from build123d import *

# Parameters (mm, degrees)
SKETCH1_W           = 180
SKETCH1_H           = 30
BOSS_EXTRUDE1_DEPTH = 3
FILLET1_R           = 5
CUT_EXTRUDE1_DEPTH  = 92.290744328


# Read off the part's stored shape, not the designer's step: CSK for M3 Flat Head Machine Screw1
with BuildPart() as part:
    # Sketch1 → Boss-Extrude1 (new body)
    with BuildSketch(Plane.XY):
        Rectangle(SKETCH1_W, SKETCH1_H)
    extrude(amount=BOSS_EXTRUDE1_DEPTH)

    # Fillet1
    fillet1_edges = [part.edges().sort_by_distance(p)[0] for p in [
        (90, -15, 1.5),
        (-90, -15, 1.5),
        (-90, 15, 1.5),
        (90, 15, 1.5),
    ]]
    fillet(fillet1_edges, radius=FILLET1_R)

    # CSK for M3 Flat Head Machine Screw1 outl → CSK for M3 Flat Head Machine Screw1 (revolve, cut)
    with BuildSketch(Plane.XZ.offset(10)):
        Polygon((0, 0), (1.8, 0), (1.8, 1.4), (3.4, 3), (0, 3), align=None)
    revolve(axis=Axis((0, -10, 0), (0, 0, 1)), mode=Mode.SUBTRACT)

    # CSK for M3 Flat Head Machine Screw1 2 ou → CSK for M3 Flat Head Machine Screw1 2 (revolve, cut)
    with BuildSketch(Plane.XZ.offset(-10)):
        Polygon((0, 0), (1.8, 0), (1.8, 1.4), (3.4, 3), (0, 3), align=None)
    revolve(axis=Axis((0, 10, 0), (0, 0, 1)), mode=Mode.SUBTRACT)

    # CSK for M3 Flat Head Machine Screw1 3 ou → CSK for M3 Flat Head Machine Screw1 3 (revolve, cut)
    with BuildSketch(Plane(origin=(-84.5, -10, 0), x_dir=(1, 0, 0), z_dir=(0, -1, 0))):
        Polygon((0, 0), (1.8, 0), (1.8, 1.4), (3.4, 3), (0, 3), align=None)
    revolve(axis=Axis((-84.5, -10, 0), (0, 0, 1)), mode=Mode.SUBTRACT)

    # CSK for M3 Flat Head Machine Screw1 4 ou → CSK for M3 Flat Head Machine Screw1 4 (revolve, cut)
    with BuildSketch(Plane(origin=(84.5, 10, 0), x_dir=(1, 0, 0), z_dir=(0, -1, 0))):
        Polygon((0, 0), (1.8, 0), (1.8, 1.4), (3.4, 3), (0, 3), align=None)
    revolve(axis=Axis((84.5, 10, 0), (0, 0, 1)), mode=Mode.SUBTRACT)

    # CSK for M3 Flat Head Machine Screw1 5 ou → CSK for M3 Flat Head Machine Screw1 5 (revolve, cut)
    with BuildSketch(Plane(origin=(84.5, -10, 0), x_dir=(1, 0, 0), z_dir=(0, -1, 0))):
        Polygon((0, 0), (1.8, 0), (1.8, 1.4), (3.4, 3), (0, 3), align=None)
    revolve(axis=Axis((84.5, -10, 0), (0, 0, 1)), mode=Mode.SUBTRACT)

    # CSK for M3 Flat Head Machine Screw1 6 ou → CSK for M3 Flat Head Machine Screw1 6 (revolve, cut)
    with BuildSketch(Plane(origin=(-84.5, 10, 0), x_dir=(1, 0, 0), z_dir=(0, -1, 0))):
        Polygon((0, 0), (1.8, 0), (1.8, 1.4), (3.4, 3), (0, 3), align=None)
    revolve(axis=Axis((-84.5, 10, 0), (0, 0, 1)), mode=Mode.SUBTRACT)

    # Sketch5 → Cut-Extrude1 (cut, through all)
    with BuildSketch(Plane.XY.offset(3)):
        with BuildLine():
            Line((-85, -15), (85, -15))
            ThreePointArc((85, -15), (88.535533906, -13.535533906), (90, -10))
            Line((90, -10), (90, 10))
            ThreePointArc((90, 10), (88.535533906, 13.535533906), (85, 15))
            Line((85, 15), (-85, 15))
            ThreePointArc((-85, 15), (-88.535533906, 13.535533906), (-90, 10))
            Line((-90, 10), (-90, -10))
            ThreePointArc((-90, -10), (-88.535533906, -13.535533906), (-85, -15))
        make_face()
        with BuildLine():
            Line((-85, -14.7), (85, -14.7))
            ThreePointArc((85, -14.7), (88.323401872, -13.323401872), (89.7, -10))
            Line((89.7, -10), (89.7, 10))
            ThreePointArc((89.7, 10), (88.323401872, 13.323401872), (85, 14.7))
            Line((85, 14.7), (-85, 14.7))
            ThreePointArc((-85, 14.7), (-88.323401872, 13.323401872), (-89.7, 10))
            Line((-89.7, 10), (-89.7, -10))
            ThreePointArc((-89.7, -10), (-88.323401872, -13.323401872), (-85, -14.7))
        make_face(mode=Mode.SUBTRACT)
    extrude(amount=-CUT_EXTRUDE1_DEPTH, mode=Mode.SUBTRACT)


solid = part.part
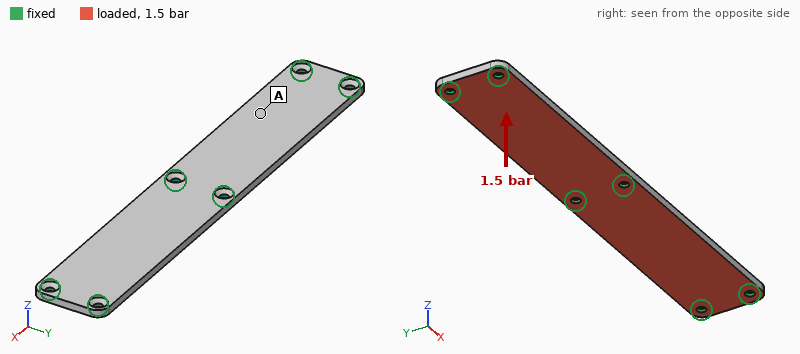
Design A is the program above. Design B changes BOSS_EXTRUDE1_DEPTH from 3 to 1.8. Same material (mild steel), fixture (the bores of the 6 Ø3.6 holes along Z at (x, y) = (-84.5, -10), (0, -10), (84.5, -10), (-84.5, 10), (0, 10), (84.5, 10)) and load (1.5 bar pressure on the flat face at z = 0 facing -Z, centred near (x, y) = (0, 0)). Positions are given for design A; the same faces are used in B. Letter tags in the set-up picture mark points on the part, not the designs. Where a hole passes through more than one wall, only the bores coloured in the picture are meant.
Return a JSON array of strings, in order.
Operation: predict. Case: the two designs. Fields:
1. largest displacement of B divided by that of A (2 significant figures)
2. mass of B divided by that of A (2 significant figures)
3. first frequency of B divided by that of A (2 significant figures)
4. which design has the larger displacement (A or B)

["3.8", "0.60", "0.70", "B"]
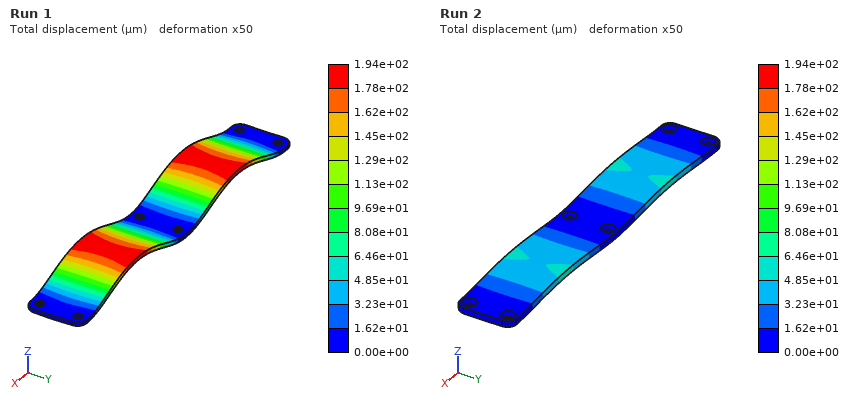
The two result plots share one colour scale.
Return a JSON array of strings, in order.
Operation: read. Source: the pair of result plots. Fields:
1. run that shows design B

["Run 1"]
